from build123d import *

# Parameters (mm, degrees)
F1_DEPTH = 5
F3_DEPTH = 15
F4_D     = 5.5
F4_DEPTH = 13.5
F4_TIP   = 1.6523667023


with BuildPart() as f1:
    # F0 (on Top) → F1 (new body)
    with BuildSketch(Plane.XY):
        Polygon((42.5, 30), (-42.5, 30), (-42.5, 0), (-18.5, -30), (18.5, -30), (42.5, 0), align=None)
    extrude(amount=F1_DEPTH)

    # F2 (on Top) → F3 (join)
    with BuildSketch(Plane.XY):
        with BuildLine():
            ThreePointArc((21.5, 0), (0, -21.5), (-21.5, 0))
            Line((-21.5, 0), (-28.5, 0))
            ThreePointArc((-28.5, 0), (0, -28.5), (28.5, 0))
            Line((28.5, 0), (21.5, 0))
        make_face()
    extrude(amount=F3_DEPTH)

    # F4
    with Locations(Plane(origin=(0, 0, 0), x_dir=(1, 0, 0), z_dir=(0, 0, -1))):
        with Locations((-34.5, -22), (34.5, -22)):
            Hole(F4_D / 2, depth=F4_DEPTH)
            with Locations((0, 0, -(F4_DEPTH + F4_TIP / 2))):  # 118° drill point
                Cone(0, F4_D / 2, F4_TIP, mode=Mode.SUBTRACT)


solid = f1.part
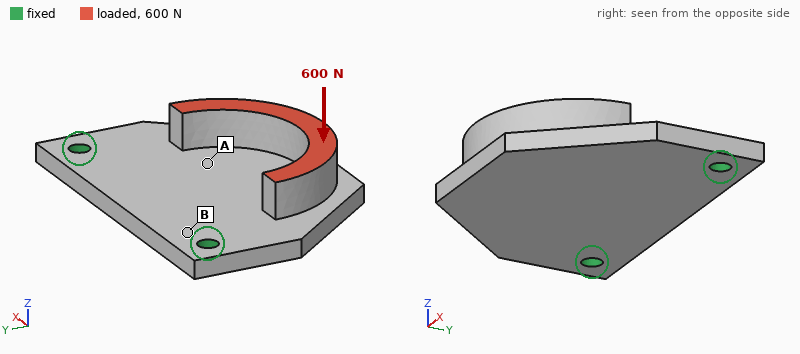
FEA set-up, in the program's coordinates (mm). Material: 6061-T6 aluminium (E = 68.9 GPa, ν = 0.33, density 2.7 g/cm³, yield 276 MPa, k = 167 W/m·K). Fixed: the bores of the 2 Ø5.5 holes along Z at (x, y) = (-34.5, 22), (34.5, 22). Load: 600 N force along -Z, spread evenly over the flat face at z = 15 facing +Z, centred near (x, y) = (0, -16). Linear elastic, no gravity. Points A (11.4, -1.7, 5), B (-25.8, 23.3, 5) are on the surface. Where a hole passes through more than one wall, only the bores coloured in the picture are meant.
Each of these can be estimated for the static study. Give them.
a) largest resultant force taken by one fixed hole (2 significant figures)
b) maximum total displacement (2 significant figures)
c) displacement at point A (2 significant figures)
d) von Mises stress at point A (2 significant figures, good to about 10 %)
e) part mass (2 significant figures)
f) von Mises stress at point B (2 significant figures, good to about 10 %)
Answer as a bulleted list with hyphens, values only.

- 300 N
- 0.42 mm
- 0.15 mm
- 22 MPa
- 73 g
- 55 MPa
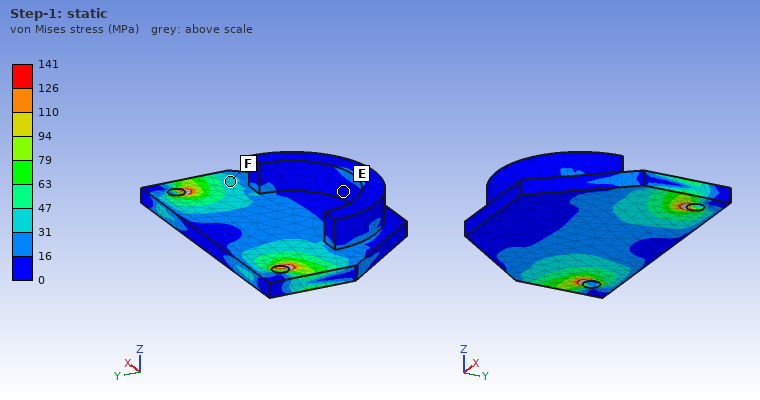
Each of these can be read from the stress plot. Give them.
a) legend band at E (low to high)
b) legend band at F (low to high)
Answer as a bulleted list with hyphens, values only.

- 0 to 16 MPa
- 31 to 47 MPa
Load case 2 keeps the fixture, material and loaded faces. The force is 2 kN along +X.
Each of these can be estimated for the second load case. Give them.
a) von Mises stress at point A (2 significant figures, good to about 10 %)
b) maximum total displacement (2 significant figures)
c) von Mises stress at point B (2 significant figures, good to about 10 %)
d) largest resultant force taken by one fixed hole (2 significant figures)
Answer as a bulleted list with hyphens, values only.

- 27 MPa
- 86 µm
- 13 MPa
- 1.5 kN
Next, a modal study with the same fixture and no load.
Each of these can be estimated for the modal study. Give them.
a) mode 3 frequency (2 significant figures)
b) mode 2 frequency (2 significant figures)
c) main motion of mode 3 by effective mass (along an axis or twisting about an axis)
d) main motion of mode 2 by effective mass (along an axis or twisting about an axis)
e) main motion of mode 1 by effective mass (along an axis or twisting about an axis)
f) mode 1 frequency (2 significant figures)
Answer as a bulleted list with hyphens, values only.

- 5800 Hz
- 4400 Hz
- along Z
- twisting about Y
- along Z
- 1200 Hz
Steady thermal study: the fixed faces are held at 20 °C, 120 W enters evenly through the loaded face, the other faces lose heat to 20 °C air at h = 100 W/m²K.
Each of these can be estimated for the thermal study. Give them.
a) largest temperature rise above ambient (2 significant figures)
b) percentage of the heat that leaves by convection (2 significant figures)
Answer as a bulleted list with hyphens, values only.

- 77 K
- 36 %
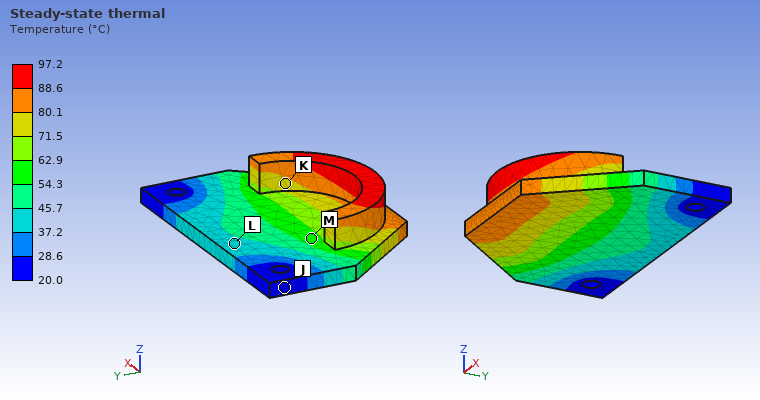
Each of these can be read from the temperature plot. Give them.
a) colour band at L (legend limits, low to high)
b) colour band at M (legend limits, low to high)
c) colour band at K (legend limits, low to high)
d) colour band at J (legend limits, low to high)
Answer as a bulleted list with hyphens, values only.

- 37.2 to 45.7 °C
- 54.3 to 62.9 °C
- 71.5 to 80.1 °C
- 20.0 to 28.6 °C
